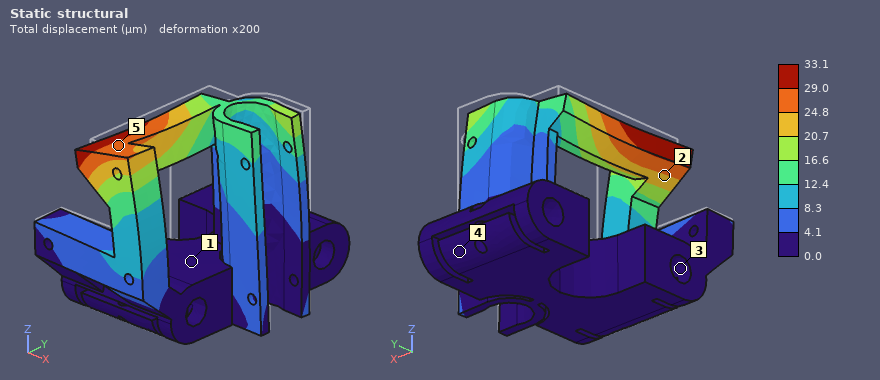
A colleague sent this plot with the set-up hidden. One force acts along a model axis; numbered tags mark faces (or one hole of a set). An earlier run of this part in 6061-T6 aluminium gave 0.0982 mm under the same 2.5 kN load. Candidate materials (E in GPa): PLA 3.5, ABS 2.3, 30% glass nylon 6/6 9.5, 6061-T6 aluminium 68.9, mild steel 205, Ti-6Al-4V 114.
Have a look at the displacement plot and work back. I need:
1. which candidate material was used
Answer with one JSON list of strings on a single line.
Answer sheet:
["mild steel"]
